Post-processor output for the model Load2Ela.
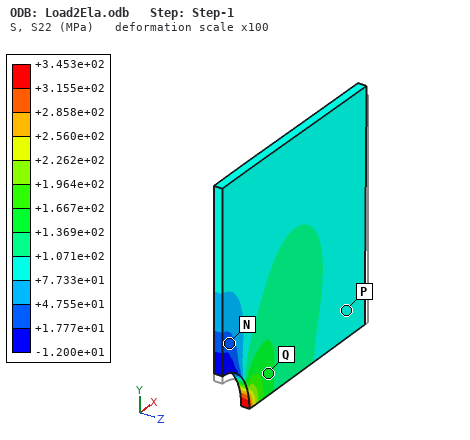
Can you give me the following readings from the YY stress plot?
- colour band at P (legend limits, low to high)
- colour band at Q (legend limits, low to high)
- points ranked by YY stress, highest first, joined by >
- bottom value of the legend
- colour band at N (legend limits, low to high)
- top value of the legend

+7.733e+01 to +1.071e+02 MPa
+1.369e+02 to +1.667e+02 MPa
Q > P > N
-1.200e+01 MPa
+1.777e+01 to +4.755e+01 MPa
+3.453e+02 MPa
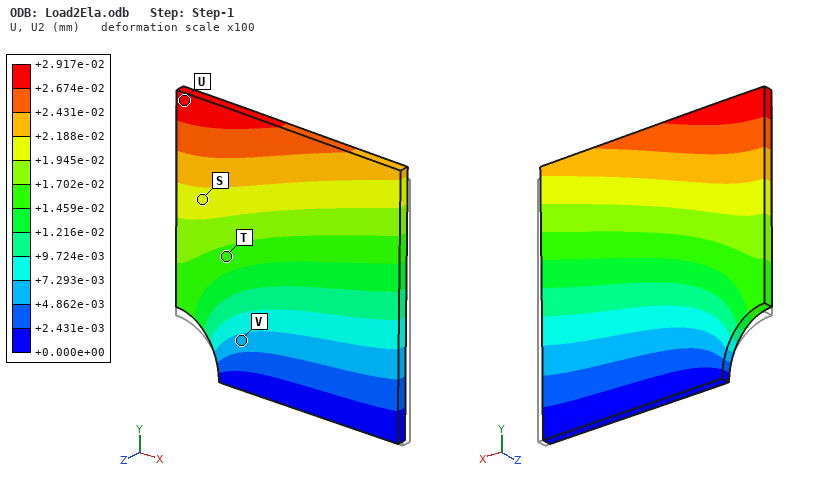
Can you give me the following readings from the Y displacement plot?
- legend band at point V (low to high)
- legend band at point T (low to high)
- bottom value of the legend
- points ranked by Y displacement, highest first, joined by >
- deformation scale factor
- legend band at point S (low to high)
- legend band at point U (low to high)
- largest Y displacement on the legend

+4.862e-03 to +7.293e-03 mm
+1.459e-02 to +1.702e-02 mm
+0.000e+00 mm
U > S > T > V
100
+1.945e-02 to +2.188e-02 mm
+2.674e-02 to +2.917e-02 mm
+2.917e-02 mm
